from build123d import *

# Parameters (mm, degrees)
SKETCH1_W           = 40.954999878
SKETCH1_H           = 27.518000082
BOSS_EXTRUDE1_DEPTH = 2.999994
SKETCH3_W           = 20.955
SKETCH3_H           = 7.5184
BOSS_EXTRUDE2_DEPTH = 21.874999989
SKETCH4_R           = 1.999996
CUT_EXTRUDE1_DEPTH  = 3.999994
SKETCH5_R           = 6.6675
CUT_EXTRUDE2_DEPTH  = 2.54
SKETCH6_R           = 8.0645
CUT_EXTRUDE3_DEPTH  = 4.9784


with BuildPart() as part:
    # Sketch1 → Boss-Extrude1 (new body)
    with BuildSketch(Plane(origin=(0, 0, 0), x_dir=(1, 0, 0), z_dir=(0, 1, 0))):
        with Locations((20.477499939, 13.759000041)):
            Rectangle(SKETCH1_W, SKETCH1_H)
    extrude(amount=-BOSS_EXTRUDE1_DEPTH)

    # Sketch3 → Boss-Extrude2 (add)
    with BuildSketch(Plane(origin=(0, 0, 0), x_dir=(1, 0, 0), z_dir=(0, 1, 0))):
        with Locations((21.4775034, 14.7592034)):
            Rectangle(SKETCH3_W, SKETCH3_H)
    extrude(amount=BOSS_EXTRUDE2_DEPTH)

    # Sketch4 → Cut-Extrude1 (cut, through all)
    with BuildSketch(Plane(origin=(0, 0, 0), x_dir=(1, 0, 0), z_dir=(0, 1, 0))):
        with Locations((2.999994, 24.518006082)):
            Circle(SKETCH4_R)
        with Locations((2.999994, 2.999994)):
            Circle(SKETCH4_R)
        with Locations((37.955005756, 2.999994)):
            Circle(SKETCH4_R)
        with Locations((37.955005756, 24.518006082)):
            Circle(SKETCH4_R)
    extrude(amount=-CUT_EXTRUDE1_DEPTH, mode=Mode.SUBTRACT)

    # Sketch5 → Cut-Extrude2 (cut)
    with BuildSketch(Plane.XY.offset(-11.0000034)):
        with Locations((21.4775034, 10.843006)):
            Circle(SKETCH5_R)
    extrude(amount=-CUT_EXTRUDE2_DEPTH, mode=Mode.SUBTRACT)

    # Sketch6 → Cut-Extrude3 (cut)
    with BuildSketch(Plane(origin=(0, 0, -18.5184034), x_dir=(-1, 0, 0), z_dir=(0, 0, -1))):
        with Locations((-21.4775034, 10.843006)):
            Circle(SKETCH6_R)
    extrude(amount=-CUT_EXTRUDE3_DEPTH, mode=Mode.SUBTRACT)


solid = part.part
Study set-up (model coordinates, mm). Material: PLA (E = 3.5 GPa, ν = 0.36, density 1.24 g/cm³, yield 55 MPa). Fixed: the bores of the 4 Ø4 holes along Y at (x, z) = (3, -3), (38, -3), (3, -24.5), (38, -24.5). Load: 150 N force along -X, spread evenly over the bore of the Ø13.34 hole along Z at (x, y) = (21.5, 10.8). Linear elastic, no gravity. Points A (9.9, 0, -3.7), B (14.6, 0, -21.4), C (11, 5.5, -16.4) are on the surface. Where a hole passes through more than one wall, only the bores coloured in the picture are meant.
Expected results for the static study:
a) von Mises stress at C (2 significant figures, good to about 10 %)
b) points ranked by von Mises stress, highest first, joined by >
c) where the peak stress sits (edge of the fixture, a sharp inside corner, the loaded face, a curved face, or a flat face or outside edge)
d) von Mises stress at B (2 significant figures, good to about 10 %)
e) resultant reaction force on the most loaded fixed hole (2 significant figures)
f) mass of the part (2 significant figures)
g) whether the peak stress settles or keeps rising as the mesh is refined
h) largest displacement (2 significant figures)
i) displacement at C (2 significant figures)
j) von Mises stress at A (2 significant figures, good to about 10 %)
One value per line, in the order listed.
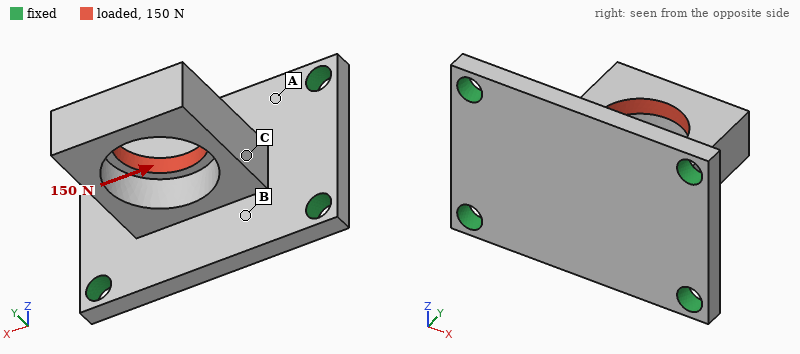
8.3 MPa
C > B > A
edge of the fixture
4.9 MPa
60 N
6.6 g
keeps rising
0.20 mm
0.071 mm
2.5 MPa
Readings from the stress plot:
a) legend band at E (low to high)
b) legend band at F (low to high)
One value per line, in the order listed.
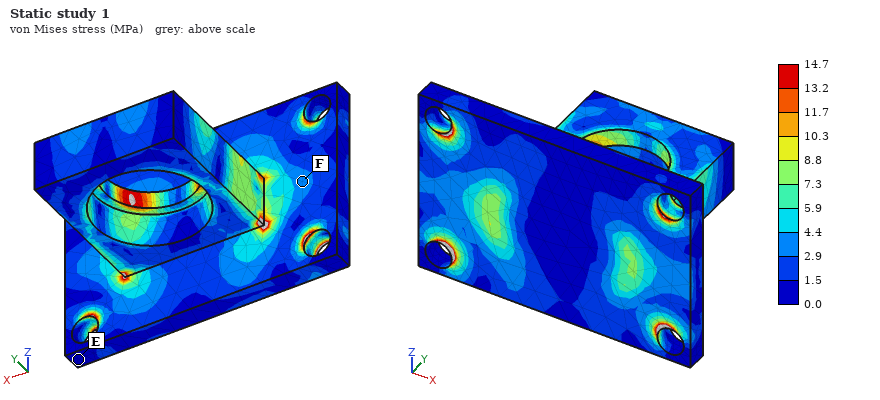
0.0 to 1.5 MPa
2.9 to 4.4 MPa
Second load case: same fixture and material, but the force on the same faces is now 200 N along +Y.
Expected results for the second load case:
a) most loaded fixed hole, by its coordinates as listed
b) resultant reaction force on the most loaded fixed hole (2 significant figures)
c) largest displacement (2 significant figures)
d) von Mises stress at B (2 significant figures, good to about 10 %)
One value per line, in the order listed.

(38, -3)
64 N
0.20 mm
3.3 MPa
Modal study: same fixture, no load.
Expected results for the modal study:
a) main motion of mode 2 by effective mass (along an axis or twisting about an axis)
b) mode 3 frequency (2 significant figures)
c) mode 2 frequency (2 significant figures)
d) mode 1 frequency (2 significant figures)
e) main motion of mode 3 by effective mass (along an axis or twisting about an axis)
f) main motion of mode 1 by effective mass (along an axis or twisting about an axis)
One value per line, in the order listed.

along X
3600 Hz
2900 Hz
2000 Hz
along Y
along Z
